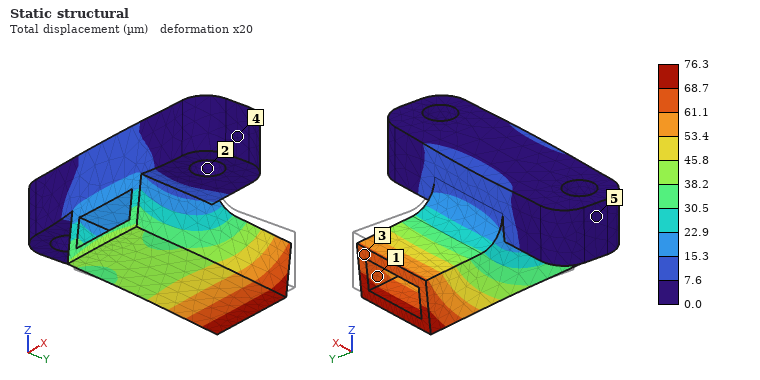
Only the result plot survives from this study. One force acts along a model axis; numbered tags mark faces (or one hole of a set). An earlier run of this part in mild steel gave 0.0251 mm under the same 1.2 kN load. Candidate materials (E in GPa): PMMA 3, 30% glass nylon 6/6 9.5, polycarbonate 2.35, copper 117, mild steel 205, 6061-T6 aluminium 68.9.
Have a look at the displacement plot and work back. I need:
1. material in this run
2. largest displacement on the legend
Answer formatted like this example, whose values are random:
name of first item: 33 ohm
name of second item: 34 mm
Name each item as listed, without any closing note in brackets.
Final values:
material in this run: 6061-T6 aluminium
largest displacement on the legend: 76.3 µm
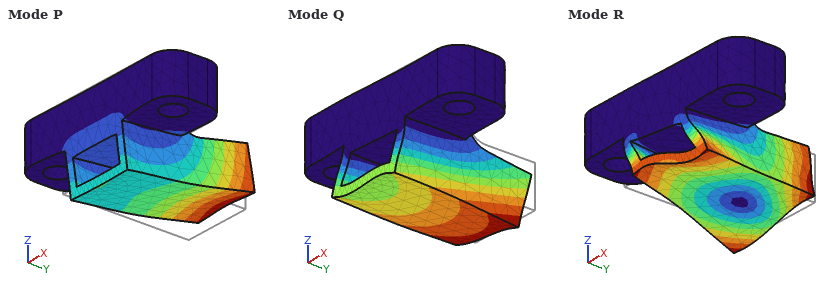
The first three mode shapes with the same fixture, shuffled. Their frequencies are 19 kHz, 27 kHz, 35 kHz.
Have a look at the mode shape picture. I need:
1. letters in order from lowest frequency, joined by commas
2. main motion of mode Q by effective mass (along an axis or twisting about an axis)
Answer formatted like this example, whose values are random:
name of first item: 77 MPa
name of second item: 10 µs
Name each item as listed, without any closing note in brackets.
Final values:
letters in order from lowest frequency, joined by commas: P, Q, R
main motion of mode Q by effective mass: along X
